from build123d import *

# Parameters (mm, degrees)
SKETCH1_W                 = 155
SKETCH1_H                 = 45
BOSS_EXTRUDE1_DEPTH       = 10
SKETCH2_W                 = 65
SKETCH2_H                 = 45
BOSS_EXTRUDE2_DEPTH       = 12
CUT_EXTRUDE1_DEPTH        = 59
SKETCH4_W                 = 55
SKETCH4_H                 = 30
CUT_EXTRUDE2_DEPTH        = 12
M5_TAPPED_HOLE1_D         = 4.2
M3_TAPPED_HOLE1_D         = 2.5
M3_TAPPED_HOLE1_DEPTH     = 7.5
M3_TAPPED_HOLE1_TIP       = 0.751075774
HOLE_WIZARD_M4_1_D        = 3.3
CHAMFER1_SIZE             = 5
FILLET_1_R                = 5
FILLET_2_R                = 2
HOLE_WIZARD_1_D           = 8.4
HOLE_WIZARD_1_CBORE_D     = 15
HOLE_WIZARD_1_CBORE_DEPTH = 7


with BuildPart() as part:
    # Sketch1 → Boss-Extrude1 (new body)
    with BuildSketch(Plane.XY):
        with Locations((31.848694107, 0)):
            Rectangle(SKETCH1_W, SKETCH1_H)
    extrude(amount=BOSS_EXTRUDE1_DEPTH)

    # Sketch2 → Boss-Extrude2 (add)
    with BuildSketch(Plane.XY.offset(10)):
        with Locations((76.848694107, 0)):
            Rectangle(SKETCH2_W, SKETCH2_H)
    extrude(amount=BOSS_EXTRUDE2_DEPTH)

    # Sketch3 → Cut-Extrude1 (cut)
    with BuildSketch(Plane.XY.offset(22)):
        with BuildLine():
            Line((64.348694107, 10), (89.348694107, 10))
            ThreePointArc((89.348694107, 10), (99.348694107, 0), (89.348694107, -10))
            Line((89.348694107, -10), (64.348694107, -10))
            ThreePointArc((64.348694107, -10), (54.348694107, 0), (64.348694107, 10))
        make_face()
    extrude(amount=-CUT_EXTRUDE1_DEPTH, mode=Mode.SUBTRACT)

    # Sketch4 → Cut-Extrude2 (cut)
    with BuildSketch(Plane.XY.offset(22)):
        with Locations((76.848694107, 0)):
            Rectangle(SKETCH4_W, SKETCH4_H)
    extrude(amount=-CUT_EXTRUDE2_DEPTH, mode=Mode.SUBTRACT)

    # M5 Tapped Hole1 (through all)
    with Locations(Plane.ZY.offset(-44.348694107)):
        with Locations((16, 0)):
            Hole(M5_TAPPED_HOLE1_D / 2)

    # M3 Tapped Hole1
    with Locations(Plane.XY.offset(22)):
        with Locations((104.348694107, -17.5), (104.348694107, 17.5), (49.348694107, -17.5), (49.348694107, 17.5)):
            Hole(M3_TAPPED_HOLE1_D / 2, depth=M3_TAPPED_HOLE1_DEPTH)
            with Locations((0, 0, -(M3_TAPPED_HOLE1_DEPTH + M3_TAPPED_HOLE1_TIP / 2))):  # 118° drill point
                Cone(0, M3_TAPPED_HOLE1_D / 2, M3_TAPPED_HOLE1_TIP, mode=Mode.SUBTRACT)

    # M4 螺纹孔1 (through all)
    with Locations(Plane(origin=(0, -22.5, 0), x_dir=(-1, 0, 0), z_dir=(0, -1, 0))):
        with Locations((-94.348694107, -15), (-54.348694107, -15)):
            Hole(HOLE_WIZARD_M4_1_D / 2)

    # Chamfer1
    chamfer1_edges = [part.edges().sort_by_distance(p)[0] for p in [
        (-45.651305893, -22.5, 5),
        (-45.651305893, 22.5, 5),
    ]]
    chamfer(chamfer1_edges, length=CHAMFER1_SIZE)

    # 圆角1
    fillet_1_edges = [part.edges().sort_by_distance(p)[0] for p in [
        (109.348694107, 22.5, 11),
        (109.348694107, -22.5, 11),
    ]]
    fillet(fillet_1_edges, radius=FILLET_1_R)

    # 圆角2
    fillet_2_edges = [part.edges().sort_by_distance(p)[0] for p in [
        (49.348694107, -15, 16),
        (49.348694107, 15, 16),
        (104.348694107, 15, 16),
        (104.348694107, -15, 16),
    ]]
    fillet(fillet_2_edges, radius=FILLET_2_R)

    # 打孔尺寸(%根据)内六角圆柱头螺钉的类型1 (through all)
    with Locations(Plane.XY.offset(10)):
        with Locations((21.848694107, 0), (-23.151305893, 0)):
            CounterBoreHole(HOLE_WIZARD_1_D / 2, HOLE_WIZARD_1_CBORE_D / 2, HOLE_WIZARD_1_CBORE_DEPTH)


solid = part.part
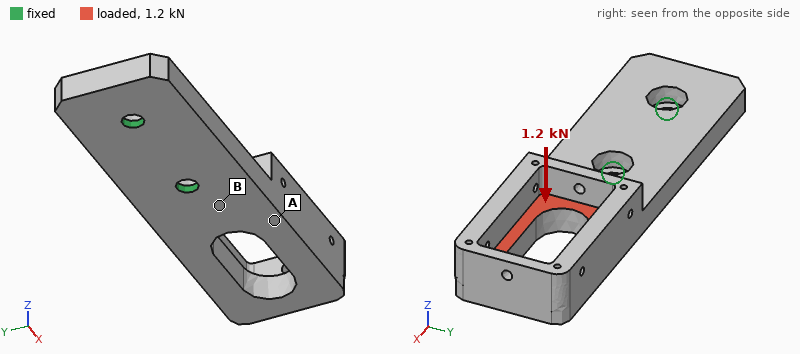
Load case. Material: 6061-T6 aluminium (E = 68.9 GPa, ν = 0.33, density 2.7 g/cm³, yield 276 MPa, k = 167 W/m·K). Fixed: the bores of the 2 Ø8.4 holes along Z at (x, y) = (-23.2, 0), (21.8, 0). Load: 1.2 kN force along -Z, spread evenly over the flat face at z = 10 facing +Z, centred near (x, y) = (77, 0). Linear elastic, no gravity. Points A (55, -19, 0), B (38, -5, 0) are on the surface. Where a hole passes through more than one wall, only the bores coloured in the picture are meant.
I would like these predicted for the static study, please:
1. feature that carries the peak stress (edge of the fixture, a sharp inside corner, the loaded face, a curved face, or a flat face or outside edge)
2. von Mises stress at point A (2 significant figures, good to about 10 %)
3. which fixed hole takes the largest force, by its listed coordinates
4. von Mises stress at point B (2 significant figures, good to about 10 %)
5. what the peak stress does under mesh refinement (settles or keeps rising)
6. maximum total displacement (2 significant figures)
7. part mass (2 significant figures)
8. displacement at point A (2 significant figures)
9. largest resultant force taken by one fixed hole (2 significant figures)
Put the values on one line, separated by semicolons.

edge of the fixture; 21 MPa; (21.8, 0); 56 MPa; keeps rising; 0.68 mm; 200 g; 0.20 mm; 3.7 kN
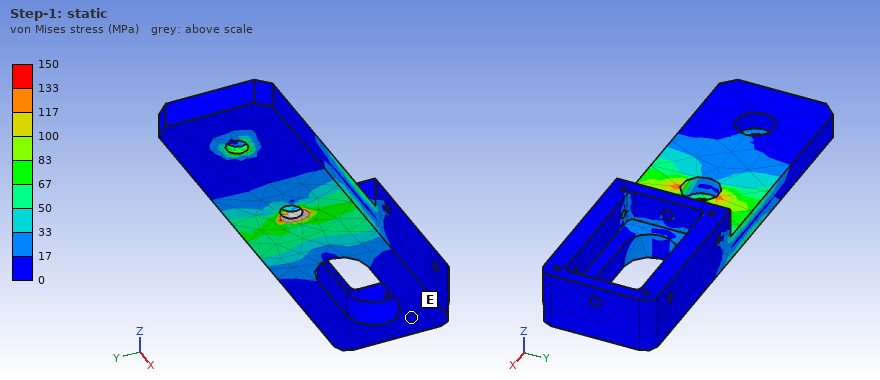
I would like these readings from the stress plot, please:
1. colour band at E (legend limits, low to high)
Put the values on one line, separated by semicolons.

0 to 17 MPa
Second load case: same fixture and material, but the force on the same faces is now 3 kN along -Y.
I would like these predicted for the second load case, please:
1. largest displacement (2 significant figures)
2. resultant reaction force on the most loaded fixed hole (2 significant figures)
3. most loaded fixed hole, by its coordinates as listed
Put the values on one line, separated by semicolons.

0.35 mm; 6.0 kN; (21.8, 0)
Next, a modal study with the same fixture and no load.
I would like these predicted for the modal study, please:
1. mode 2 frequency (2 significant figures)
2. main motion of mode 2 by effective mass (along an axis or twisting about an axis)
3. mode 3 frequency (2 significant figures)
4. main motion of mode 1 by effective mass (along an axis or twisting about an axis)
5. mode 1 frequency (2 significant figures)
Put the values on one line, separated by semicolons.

1700 Hz; along Y; 2400 Hz; along Z; 810 Hz
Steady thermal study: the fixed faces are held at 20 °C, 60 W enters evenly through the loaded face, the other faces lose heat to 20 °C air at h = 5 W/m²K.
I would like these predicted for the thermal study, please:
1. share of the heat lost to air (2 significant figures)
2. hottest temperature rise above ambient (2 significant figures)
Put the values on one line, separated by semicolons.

5.0 %; 57 K
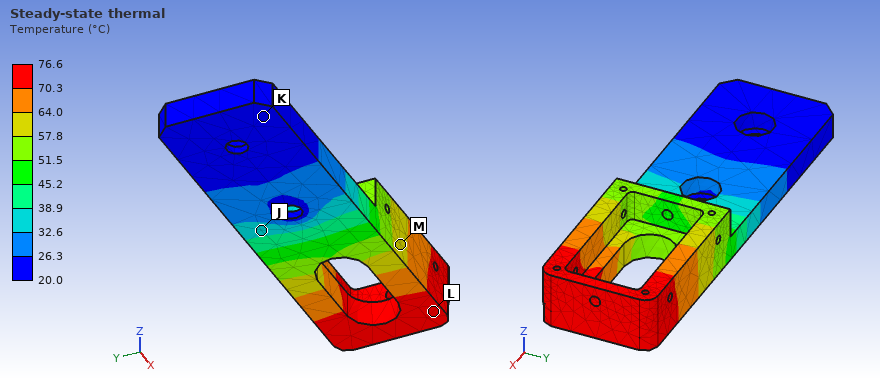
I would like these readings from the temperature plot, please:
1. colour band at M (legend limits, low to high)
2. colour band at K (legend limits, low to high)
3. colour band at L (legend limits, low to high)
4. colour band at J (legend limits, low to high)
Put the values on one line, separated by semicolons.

57.8 to 64.0 °C; 20.0 to 26.3 °C; 70.3 to 76.6 °C; 32.6 to 38.9 °C
